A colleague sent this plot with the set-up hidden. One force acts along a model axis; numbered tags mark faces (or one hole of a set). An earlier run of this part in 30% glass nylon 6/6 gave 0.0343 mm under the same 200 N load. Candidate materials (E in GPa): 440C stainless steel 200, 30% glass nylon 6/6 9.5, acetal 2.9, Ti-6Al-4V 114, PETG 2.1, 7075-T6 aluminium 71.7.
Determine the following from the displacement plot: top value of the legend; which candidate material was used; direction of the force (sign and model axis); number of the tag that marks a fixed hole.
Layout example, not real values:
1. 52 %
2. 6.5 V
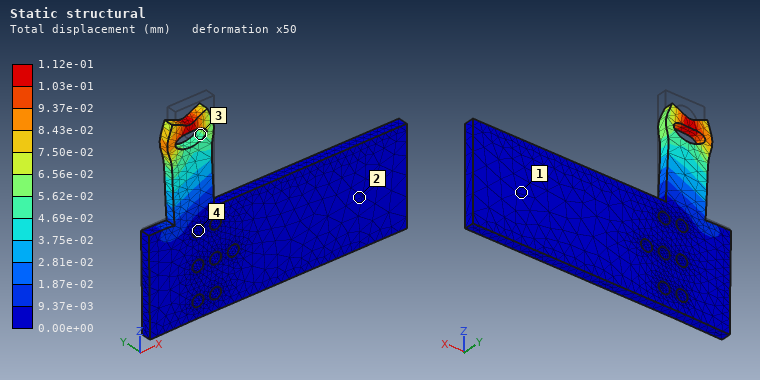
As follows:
1. 1.12e-01 mm
2. acetal
3. -Z
4. 4
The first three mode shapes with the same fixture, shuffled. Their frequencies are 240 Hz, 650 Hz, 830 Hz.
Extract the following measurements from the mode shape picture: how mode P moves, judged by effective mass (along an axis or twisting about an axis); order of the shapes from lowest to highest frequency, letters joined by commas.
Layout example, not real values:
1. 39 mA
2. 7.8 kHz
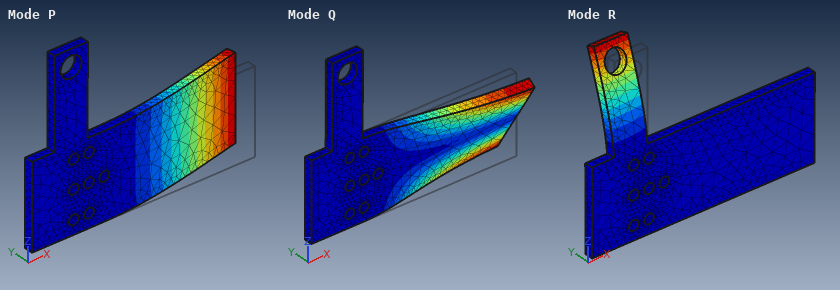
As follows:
1. along Y
2. P, R, Q
